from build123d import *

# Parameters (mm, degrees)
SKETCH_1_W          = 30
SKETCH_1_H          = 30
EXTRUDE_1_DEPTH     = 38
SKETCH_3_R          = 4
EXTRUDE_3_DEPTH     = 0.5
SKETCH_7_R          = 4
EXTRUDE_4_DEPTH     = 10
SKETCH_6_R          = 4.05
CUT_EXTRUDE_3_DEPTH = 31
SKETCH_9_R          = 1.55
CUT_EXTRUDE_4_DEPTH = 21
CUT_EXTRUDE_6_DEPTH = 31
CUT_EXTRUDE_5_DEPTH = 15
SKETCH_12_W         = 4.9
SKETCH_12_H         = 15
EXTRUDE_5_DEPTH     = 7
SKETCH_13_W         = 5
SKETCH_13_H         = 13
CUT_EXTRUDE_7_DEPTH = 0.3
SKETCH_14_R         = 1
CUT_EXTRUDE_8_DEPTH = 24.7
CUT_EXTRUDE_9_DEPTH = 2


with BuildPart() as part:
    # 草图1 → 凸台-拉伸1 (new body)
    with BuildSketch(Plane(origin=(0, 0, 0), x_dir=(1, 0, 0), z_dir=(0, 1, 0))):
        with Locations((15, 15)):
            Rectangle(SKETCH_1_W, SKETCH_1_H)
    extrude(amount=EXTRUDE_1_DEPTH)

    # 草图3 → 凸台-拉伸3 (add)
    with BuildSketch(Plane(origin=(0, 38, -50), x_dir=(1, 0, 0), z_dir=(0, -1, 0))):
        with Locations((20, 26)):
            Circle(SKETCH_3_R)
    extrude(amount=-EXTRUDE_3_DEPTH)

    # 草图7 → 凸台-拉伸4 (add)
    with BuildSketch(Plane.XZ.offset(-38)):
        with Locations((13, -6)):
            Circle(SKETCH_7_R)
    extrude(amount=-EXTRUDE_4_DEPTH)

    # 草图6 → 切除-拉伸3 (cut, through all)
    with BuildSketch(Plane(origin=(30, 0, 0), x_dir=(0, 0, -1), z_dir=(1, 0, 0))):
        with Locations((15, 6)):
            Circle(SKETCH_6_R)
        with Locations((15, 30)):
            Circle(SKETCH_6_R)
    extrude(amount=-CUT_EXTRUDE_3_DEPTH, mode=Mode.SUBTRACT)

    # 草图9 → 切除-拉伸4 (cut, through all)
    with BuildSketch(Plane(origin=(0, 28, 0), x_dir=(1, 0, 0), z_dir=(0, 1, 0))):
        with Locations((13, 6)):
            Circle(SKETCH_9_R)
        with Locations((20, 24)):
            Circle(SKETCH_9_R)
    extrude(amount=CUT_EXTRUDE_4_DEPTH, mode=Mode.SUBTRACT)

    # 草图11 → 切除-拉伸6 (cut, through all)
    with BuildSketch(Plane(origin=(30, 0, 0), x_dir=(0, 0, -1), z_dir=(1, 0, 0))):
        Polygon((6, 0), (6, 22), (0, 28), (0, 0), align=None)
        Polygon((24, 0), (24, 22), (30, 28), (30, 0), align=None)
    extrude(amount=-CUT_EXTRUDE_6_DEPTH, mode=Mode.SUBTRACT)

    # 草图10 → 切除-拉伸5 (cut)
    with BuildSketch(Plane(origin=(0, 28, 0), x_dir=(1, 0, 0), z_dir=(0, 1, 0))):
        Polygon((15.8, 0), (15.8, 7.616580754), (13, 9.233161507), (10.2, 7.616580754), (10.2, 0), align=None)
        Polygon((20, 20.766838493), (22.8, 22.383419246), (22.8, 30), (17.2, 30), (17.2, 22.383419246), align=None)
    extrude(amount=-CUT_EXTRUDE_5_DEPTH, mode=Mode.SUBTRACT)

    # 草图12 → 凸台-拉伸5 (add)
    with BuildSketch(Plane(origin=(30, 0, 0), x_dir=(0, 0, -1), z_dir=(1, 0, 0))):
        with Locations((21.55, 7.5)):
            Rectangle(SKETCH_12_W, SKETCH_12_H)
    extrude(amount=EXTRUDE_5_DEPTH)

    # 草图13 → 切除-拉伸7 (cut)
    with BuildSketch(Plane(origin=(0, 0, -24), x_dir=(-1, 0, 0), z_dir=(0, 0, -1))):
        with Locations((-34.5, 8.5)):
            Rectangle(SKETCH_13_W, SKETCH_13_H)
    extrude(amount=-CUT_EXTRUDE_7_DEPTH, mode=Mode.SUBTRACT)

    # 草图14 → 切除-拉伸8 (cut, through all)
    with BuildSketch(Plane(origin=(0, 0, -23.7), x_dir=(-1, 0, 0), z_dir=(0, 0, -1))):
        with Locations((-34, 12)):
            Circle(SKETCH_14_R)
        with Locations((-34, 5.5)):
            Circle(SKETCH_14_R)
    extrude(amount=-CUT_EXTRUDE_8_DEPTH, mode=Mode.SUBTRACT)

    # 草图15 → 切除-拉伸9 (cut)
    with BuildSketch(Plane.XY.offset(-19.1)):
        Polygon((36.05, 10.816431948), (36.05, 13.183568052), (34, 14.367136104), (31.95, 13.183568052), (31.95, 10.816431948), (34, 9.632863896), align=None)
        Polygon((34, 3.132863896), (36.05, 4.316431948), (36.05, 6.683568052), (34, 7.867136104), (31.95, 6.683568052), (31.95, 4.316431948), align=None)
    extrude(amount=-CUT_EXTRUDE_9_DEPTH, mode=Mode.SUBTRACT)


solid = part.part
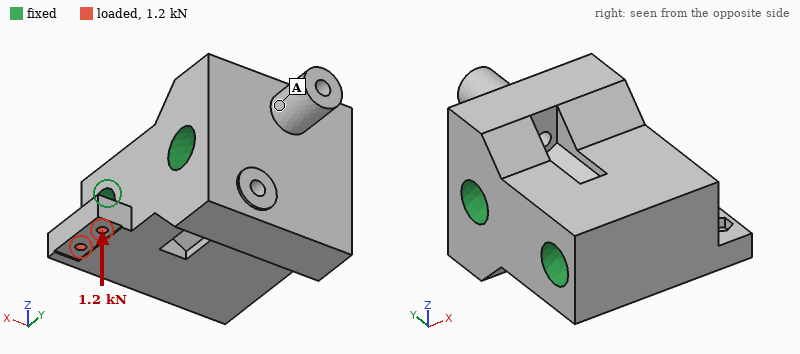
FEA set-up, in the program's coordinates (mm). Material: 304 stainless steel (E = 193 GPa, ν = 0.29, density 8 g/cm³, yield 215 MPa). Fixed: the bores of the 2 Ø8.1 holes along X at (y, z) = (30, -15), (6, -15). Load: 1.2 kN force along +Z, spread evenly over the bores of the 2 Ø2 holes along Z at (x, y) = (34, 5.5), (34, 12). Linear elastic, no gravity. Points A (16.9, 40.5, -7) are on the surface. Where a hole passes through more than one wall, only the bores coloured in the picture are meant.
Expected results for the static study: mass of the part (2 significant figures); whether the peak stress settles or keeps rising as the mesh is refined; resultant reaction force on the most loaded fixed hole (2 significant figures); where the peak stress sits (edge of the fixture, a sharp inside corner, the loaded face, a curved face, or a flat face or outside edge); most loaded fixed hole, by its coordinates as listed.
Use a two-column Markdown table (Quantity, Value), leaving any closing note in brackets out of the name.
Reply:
| Quantity | Value |
|---|---|
| mass of the part | 180 g |
| whether the peak stress settles or keeps rising as the mesh is refined | keeps rising |
| resultant reaction force on the most loaded fixed hole | 1.1 kN |
| where the peak stress sits | edge of the fixture |
| most loaded fixed hole, by its coordinates as listed | (6, -15) |
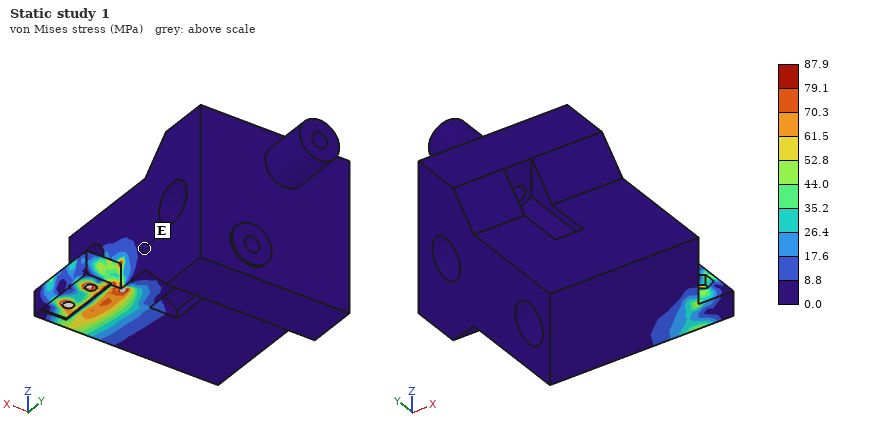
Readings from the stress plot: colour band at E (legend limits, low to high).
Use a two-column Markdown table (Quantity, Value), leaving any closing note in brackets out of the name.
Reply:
| Quantity | Value |
|---|---|
| colour band at E | 0.0 to 8.8 MPa |
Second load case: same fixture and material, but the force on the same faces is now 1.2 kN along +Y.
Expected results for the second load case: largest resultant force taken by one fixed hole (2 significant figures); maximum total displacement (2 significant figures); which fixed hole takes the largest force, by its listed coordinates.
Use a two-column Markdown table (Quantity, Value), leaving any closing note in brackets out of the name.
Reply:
| Quantity | Value |
|---|---|
| largest resultant force taken by one fixed hole | 940 N |
| maximum total displacement | 4.2 µm |
| which fixed hole takes the largest force, by its listed coordinates | (6, -15) |
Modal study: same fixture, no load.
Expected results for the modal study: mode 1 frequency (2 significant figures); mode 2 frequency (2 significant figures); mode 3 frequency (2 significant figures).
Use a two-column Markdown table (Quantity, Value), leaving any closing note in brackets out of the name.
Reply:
| Quantity | Value |
|---|---|
| mode 1 frequency | 30 kHz |
| mode 2 frequency | 32 kHz |
| mode 3 frequency | 40 kHz |
